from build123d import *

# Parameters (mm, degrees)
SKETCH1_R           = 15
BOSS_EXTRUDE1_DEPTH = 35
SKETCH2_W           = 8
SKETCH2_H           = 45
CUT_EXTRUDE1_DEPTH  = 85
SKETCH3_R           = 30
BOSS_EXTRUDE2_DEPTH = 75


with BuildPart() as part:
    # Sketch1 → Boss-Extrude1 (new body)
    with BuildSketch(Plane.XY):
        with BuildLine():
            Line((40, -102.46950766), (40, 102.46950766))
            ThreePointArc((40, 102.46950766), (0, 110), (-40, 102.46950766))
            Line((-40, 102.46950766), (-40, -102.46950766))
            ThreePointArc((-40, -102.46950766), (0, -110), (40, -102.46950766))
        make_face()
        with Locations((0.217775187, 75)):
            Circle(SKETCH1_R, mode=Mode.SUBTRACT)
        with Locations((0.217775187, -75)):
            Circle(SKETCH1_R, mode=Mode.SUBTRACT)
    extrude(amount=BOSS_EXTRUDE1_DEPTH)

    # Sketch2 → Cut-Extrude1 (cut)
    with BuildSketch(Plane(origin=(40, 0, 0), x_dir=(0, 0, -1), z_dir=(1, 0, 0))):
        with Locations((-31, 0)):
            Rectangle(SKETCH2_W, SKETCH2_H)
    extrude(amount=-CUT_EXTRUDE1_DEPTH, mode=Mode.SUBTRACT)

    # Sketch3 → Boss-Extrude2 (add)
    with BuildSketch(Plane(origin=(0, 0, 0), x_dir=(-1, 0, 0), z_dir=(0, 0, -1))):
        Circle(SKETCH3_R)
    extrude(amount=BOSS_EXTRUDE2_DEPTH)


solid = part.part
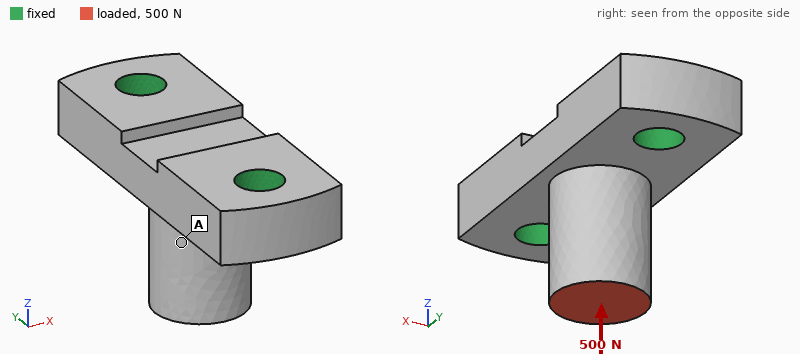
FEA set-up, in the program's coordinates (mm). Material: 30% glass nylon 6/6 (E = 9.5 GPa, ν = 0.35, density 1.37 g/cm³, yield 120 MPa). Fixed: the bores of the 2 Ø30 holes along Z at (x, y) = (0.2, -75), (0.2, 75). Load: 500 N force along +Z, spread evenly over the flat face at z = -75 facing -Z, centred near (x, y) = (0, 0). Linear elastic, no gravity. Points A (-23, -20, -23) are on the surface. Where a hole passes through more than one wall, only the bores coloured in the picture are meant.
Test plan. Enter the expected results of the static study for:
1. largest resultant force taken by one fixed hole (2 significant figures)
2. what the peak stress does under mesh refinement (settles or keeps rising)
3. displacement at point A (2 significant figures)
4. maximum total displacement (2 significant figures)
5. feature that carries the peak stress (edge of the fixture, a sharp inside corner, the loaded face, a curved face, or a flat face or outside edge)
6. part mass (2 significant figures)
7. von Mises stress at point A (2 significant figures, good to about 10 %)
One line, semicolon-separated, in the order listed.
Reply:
280 N; keeps rising; 3.6 µm; 4.6 µm; edge of the fixture; 1.0 kg; 0.16 MPa
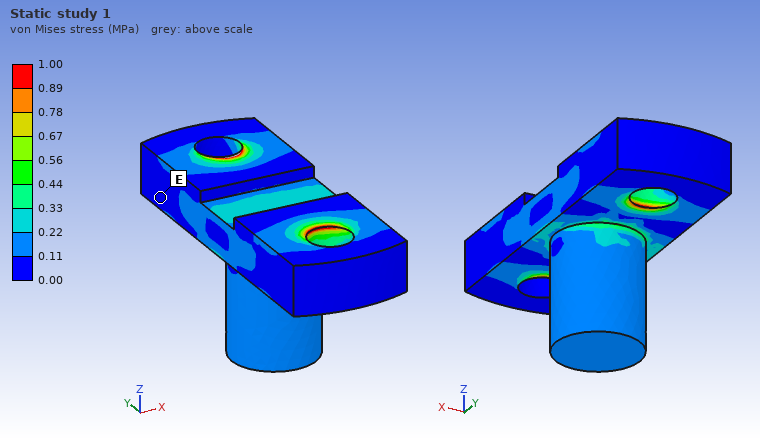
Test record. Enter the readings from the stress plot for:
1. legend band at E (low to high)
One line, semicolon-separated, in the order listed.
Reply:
0.00 to 0.11 MPa
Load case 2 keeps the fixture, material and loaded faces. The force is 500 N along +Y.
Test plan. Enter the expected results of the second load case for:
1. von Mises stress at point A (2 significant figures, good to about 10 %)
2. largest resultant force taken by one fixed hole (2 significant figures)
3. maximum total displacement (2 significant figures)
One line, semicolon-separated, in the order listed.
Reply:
0.81 MPa; 520 N; 32 µm
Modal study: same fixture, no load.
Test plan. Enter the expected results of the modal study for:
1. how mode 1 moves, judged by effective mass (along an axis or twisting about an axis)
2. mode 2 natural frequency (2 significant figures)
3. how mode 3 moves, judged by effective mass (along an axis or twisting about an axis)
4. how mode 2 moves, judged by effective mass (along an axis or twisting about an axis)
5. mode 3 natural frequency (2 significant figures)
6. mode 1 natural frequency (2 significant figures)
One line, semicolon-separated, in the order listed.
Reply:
along X; 2000 Hz; along Z; along Y; 2700 Hz; 1300 Hz
